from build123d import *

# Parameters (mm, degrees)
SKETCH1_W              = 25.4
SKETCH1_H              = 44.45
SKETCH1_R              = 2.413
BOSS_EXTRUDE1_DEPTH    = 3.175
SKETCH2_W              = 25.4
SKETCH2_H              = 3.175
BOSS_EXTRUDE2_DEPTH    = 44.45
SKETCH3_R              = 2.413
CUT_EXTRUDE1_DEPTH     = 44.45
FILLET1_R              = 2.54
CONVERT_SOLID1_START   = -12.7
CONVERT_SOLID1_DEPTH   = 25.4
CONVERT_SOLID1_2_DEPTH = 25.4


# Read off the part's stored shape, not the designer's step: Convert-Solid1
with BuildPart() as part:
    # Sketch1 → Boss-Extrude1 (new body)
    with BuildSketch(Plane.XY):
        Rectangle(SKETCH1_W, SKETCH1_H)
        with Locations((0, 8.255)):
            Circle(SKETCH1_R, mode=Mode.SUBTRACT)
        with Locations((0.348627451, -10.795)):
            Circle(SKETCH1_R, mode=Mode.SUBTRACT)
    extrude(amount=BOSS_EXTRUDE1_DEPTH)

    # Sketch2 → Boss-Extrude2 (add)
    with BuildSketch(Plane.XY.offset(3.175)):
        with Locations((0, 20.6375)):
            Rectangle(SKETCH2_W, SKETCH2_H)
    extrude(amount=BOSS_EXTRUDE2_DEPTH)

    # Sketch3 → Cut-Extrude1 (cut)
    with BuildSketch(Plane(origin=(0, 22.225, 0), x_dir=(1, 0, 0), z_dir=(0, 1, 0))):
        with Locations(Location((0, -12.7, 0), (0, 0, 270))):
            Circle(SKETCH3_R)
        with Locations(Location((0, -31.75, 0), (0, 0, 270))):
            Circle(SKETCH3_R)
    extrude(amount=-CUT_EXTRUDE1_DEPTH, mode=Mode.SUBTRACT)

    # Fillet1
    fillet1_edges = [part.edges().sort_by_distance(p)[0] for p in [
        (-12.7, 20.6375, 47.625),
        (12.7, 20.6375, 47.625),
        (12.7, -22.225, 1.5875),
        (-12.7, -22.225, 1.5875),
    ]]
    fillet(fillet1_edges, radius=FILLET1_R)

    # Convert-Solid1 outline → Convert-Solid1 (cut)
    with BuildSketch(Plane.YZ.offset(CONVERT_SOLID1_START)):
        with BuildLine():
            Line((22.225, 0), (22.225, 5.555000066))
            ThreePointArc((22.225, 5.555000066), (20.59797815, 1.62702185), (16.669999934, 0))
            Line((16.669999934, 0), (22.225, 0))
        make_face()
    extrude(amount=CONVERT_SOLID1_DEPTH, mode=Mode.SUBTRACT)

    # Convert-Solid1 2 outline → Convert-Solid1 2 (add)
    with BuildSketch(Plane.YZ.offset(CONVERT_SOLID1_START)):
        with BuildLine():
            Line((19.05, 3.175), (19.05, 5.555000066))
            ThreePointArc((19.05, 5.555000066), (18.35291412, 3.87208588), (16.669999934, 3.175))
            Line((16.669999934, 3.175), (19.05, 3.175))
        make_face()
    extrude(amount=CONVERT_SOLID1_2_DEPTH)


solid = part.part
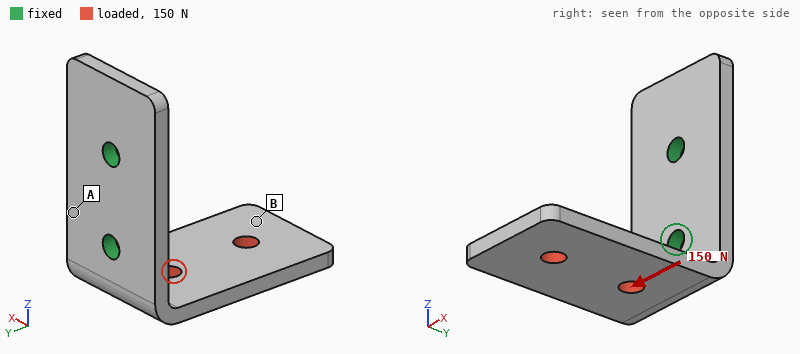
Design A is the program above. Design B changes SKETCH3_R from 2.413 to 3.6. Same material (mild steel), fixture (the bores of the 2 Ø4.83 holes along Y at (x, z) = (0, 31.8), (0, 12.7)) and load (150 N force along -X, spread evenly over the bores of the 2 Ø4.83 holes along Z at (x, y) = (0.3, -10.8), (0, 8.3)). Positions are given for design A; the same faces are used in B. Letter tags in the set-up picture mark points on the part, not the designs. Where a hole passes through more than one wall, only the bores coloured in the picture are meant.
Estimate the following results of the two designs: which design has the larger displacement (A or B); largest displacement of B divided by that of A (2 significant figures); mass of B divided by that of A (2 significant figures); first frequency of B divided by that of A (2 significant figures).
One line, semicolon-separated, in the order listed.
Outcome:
A; 0.76; 0.98; 1.0
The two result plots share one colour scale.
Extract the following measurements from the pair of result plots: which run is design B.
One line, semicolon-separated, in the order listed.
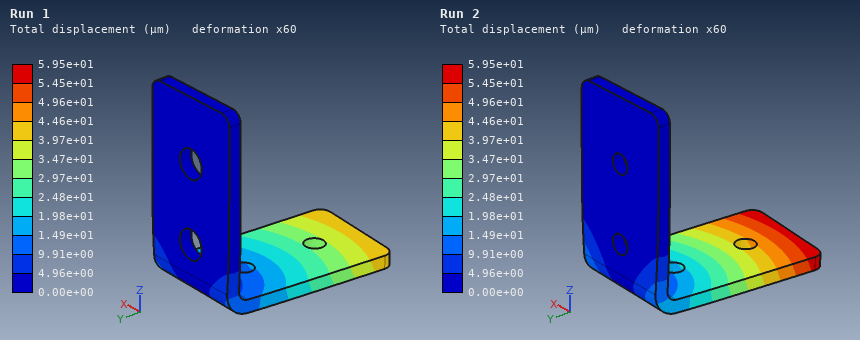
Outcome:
Run 1
